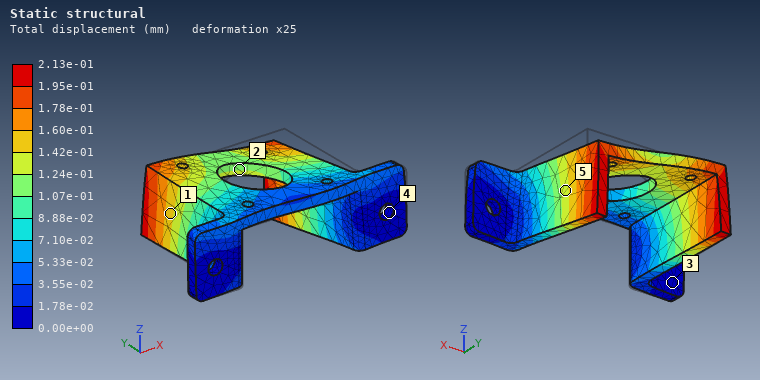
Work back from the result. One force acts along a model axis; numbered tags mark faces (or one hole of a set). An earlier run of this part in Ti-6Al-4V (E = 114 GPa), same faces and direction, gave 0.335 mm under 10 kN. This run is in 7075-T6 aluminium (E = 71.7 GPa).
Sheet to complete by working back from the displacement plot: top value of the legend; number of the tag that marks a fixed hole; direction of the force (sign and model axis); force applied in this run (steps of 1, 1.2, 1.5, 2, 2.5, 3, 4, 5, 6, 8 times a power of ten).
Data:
2.13e-01 mm
4
-X
4 kN
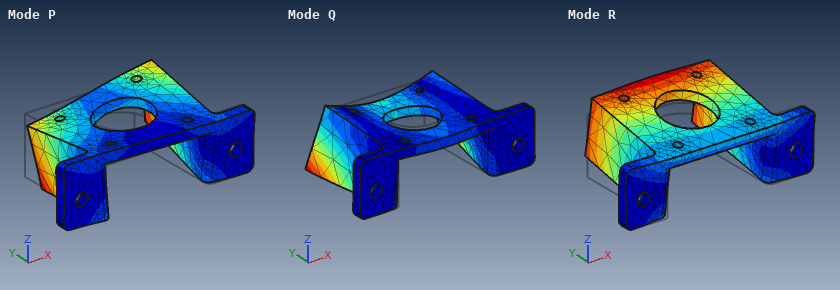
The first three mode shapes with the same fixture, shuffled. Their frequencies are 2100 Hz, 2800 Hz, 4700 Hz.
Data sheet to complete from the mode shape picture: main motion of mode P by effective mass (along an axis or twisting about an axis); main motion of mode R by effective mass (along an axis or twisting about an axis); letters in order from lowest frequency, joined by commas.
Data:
along X
along Z
R, P, Q
